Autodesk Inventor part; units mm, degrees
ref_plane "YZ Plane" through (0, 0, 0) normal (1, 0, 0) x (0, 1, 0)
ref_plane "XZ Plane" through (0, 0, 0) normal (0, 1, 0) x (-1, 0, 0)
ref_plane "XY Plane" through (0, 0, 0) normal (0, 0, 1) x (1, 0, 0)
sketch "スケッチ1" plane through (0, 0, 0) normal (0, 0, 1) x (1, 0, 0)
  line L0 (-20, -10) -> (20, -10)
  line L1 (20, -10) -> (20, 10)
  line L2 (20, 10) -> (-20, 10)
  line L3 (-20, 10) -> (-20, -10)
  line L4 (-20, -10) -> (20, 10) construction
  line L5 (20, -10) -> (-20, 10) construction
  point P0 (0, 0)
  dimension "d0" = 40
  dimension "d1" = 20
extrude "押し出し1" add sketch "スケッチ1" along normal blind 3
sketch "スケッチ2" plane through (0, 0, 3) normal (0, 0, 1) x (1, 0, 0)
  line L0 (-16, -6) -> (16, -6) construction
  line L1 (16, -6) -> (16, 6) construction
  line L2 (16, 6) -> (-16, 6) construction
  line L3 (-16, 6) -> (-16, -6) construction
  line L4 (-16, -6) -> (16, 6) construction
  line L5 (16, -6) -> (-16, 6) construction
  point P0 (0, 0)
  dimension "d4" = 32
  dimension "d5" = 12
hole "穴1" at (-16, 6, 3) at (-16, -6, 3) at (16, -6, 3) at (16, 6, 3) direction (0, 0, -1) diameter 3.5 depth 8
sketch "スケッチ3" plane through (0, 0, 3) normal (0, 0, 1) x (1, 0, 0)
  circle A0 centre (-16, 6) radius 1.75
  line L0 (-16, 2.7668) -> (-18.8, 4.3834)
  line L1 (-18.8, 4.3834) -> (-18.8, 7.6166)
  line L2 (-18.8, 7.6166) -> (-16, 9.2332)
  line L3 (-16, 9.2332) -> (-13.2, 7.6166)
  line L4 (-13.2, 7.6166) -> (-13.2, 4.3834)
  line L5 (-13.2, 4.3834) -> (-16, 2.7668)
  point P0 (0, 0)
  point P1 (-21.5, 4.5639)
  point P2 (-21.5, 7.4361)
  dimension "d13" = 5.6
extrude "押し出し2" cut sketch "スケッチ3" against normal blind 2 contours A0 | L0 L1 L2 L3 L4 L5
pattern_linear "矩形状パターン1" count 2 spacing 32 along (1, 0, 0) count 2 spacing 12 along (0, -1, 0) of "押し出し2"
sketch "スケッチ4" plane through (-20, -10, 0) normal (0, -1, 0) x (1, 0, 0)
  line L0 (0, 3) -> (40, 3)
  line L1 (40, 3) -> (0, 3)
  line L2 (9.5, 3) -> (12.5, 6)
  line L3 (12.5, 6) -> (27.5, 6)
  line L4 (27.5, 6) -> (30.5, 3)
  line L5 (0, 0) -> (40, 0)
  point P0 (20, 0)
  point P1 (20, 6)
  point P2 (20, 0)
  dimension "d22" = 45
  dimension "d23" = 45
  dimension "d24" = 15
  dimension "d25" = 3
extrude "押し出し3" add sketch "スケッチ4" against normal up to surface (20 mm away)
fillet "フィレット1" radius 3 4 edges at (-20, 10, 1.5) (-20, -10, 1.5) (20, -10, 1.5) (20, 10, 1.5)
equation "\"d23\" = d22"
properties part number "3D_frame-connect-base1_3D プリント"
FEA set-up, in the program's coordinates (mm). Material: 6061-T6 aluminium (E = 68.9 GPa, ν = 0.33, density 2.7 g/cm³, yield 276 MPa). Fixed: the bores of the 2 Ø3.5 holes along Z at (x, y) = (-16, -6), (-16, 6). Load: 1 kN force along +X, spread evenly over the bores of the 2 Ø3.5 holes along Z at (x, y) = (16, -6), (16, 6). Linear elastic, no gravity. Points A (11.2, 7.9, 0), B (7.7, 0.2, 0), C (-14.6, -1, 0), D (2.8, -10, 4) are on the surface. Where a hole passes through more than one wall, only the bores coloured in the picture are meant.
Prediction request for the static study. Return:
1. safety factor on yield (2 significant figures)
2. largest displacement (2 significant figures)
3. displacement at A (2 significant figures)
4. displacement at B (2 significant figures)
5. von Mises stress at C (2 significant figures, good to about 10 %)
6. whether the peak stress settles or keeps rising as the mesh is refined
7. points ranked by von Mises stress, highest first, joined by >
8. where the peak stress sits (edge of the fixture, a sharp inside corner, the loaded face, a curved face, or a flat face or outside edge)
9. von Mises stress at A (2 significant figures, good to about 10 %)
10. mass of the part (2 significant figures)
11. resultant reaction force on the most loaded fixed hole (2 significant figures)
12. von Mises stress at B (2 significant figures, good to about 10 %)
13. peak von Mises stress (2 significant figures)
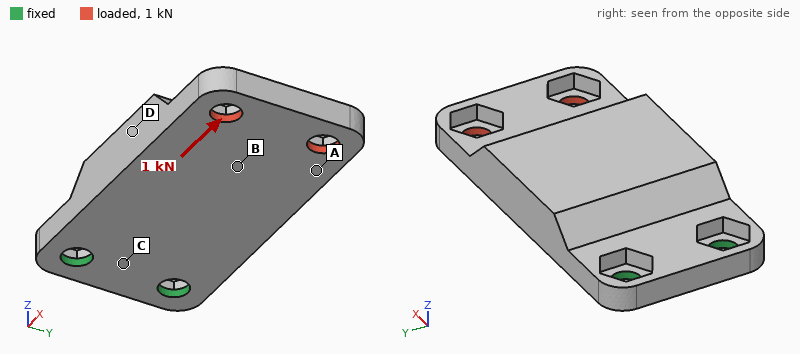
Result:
2.1
0.10 mm
0.055 mm
0.044 mm
22 MPa
settles
A > B > C > D
the loaded face
53 MPa
8.6 g
500 N
35 MPa
130 MPa
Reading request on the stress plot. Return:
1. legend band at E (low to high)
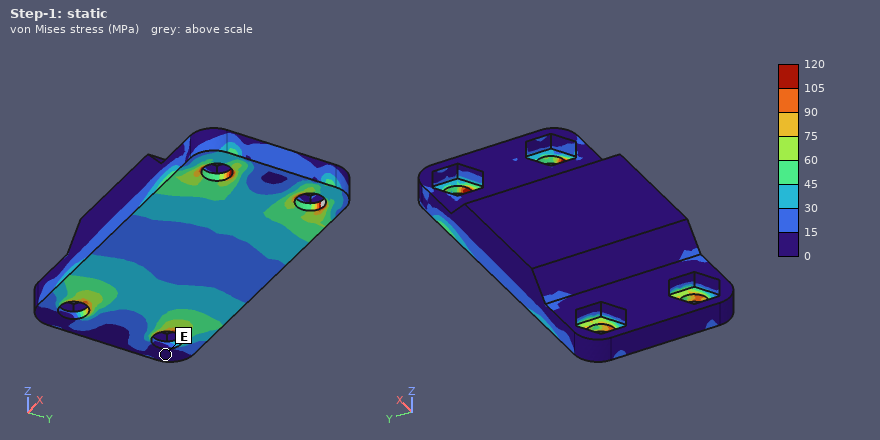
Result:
0 to 15 MPa
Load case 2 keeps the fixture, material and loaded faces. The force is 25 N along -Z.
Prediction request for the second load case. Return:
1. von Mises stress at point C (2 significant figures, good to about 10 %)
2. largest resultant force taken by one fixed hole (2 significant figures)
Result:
24 MPa
14 N
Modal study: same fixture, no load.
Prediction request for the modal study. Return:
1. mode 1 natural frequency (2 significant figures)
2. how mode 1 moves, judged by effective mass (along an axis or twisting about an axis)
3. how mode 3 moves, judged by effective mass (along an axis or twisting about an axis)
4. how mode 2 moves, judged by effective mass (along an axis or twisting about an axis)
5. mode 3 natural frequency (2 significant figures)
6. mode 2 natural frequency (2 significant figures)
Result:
1500 Hz
along Z
along Y
along Y
10 kHz
7600 Hz
